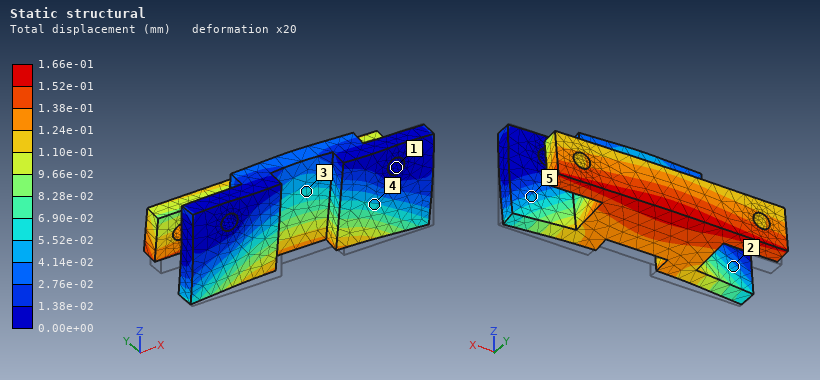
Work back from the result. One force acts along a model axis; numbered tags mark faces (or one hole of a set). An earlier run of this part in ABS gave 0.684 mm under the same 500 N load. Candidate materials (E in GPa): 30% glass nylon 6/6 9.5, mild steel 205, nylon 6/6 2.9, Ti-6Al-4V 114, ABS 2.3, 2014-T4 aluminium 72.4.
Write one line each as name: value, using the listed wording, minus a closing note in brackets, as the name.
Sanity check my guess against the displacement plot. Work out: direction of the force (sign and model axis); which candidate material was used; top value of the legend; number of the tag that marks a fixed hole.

direction of the force: +Y
which candidate material was used: 30% glass nylon 6/6
top value of the legend: 1.66e-01 mm
number of the tag that marks a fixed hole: 1
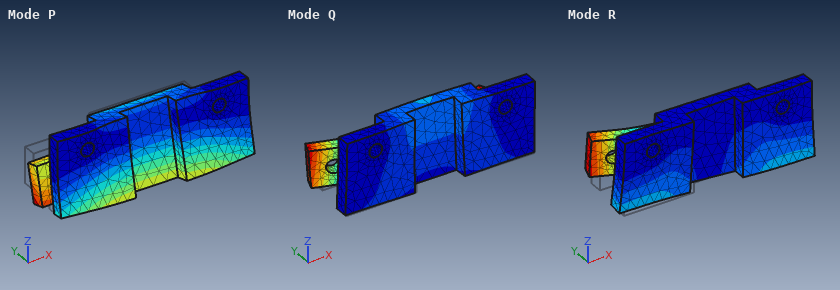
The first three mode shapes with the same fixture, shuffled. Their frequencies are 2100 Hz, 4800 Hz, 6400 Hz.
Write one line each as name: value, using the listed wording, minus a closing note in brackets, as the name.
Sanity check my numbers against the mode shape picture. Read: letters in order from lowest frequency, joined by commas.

letters in order from lowest frequency, joined by commas: P, R, Q
